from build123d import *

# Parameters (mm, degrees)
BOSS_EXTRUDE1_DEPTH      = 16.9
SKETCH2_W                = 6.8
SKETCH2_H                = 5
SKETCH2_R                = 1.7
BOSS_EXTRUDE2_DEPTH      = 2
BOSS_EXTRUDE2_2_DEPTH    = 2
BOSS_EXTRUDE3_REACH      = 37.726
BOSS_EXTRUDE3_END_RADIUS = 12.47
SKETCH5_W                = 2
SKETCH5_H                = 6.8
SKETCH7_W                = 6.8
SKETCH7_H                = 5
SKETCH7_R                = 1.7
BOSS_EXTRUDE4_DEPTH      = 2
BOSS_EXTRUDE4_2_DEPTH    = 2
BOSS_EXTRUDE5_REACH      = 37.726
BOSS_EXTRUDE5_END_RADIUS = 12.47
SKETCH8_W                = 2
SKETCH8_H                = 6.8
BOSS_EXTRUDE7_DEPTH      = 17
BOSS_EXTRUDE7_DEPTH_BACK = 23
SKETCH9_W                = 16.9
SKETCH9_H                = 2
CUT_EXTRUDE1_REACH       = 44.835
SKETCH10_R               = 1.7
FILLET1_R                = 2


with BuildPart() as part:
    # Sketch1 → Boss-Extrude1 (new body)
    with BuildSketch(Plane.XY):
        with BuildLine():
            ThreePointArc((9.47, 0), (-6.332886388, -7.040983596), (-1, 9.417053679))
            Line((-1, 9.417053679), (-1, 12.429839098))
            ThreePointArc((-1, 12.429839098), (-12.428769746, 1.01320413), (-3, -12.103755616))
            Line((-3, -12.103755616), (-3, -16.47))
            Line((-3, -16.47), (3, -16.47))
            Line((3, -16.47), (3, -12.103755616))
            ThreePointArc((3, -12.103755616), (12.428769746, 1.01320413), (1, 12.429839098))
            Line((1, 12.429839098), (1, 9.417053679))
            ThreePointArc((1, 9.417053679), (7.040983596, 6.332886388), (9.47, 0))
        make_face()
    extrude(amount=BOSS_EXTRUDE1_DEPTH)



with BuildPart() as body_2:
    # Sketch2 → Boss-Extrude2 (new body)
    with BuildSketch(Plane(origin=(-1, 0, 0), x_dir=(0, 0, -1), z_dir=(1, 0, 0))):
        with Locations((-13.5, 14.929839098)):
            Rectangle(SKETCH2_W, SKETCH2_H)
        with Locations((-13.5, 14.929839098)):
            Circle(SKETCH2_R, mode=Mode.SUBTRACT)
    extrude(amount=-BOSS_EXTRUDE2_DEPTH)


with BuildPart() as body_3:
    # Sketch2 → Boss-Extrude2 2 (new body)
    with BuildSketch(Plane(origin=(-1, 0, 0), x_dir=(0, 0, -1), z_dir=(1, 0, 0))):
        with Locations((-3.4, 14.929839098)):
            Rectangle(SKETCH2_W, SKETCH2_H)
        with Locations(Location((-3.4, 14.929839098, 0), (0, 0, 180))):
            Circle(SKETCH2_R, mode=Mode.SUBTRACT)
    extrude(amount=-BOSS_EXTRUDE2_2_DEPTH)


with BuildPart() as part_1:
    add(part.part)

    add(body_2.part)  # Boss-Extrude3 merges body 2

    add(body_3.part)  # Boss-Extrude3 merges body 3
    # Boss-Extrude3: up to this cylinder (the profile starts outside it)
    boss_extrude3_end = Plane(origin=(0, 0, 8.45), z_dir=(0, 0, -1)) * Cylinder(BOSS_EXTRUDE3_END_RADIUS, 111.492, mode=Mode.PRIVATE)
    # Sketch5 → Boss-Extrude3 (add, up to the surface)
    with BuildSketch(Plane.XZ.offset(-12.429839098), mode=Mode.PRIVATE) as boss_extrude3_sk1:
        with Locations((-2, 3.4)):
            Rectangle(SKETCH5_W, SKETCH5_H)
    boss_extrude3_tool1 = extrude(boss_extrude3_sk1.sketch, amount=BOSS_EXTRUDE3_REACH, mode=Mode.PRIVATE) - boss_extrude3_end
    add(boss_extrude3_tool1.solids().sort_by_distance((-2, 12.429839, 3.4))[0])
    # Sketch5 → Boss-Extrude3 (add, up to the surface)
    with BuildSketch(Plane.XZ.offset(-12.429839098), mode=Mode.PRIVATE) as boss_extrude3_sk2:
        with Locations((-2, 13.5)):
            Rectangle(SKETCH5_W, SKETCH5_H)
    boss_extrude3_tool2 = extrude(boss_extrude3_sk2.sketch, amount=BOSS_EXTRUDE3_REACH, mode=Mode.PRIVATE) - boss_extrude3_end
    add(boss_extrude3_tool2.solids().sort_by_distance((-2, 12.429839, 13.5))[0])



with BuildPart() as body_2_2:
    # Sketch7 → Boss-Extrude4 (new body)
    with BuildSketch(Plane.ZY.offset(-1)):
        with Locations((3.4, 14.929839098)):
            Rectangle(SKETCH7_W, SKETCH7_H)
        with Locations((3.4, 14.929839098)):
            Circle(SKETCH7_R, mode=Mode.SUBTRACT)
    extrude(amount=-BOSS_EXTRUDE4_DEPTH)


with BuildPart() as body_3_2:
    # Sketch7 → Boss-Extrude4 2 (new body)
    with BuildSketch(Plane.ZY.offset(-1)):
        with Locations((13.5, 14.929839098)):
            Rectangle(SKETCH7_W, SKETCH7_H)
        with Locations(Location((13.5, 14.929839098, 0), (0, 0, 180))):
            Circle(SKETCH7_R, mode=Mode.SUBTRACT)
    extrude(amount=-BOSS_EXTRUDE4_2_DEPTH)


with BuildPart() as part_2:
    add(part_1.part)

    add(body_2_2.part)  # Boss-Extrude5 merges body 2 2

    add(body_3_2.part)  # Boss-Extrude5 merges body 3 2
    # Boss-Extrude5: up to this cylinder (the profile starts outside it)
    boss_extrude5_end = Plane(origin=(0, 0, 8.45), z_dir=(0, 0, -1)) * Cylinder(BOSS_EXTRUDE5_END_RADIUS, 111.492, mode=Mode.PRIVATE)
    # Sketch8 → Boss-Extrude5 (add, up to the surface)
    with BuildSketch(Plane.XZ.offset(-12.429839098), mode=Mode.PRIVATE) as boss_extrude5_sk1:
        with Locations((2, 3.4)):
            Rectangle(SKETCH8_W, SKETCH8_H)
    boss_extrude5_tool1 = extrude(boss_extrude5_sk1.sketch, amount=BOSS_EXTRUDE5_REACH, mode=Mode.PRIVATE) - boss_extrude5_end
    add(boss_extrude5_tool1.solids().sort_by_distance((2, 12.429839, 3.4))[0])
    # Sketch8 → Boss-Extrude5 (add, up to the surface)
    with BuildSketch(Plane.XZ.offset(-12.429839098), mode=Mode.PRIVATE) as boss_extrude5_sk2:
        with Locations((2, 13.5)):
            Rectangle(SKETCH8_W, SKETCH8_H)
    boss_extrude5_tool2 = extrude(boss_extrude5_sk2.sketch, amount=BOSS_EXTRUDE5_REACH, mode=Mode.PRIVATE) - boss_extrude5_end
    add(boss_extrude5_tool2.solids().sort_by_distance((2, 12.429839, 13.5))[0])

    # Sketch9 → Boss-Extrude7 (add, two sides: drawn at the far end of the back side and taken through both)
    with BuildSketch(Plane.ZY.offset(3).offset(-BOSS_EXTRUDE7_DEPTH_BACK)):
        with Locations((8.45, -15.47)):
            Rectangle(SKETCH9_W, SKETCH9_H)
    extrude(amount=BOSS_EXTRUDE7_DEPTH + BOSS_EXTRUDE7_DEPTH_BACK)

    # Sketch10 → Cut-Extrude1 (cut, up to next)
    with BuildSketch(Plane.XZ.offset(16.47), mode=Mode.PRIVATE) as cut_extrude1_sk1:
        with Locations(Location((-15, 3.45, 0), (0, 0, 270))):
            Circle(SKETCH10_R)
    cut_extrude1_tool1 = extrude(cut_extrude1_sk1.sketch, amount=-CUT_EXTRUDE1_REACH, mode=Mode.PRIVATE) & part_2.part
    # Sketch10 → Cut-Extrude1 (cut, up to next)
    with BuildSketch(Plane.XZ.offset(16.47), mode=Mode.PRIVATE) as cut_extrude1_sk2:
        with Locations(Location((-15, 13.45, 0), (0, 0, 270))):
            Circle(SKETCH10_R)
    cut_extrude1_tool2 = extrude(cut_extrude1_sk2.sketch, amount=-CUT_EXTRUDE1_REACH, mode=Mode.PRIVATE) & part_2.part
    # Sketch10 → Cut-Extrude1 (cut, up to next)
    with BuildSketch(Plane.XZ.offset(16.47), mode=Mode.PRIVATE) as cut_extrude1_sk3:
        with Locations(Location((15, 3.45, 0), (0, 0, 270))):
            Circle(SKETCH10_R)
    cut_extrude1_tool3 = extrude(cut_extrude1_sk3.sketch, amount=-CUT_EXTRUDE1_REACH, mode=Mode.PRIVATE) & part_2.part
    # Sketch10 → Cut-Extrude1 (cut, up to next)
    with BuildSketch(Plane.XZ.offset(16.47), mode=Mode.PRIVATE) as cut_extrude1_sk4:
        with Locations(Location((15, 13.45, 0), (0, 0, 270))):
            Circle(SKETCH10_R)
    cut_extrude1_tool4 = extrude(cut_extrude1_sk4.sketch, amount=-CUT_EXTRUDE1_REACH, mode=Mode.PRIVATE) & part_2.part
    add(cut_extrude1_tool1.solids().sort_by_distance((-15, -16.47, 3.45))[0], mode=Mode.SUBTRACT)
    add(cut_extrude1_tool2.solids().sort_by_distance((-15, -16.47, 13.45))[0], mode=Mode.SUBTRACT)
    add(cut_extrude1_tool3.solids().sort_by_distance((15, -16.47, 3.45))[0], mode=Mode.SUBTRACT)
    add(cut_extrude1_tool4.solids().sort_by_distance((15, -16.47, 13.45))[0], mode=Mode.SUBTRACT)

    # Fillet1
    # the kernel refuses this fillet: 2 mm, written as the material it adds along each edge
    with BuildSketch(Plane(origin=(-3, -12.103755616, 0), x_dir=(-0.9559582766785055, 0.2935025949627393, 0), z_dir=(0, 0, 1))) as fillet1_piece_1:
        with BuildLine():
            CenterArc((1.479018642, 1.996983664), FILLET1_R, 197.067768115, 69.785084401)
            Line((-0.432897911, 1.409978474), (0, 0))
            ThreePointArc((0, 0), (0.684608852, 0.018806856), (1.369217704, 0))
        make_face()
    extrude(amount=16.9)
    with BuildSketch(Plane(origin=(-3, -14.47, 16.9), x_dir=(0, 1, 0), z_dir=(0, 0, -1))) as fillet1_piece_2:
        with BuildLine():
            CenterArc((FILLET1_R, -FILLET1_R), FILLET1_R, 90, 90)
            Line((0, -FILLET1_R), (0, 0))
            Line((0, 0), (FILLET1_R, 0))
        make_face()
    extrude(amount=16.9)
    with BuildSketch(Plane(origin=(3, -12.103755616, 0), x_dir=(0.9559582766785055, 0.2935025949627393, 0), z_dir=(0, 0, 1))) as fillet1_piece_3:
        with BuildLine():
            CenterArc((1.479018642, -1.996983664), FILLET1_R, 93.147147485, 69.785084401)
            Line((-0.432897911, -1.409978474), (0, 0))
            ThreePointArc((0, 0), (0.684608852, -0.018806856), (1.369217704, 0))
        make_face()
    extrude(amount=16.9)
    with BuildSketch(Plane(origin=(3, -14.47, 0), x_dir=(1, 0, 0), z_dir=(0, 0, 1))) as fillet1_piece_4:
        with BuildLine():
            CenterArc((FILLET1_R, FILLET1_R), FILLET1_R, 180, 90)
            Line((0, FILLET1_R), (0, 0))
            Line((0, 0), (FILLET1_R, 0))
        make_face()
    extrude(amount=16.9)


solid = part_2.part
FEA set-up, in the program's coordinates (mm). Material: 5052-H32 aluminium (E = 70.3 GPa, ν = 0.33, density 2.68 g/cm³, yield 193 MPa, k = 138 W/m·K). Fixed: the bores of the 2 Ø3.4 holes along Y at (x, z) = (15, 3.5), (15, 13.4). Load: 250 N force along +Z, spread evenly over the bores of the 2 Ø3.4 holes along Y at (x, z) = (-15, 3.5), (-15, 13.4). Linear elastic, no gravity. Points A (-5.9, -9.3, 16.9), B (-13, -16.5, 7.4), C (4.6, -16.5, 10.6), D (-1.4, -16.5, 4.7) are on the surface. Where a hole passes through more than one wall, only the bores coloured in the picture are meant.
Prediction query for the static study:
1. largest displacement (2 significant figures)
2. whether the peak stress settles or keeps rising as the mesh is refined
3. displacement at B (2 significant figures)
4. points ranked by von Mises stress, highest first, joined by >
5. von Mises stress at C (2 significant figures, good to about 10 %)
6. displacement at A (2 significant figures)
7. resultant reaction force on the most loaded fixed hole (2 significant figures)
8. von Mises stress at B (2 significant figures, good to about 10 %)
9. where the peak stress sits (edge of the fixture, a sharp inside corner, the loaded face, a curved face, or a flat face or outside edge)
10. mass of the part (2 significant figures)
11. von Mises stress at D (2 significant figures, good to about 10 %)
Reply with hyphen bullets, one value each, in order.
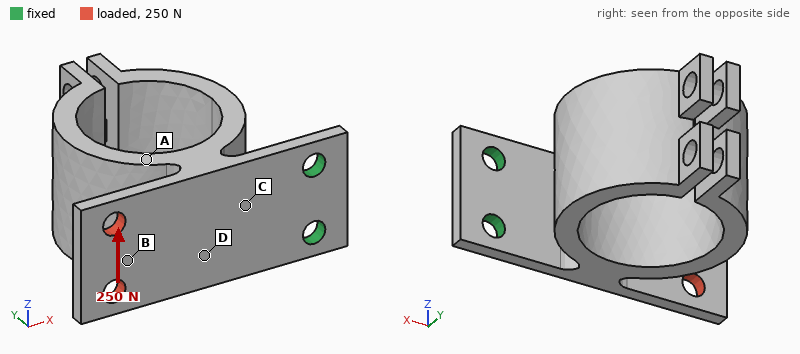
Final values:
- 58 µm
- keeps rising
- 41 µm
- C > D > B > A
- 28 MPa
- 25 µm
- 640 N
- 14 MPa
- edge of the fixture
- 14 g
- 19 MPa
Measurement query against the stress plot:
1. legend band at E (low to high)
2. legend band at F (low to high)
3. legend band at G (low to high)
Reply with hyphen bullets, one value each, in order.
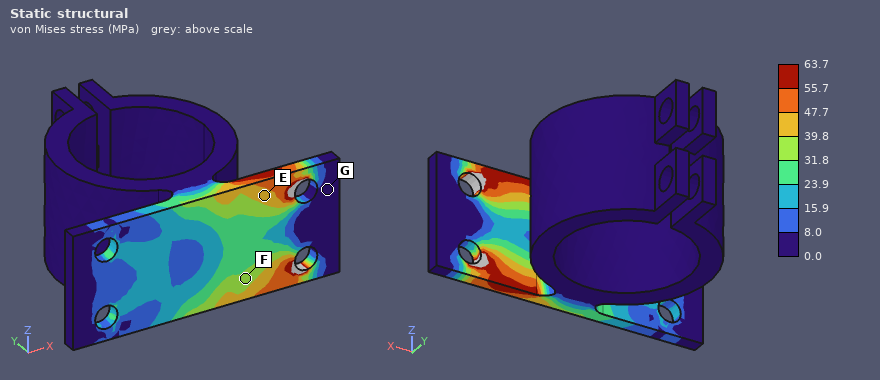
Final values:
- 39.8 to 47.7 MPa
- 31.8 to 39.8 MPa
- 0.0 to 8.0 MPa
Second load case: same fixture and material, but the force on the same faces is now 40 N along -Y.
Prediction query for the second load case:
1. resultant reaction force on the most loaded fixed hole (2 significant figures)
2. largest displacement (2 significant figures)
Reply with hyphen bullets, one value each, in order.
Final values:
- 20 N
- 0.43 mm
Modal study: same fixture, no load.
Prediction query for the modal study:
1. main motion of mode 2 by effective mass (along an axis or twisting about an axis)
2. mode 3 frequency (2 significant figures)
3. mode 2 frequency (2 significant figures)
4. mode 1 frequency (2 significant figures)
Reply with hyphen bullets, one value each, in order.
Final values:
- along Z
- 2600 Hz
- 1300 Hz
- 610 Hz
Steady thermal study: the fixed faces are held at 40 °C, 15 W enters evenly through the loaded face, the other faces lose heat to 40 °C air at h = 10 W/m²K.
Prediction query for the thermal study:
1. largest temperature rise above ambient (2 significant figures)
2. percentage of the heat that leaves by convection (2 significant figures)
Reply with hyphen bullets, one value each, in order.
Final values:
- 85 K
- 11 %
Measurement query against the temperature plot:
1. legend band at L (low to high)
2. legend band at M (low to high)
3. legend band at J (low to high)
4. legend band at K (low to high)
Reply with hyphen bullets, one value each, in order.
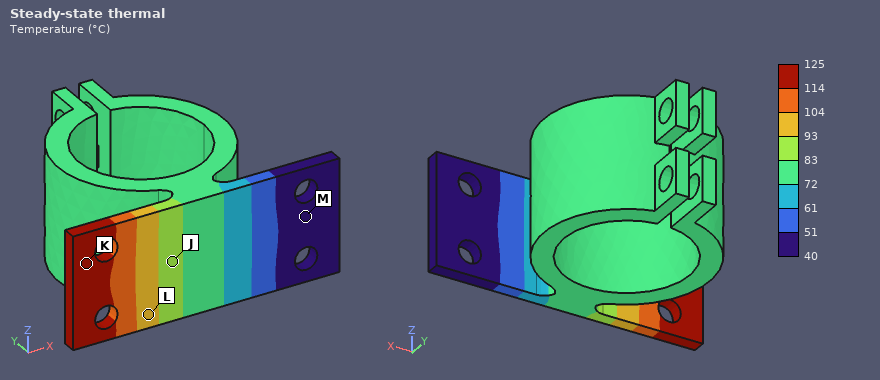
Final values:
- 93 to 104 °C
- 40 to 51 °C
- 83 to 93 °C
- 114 to 125 °C
